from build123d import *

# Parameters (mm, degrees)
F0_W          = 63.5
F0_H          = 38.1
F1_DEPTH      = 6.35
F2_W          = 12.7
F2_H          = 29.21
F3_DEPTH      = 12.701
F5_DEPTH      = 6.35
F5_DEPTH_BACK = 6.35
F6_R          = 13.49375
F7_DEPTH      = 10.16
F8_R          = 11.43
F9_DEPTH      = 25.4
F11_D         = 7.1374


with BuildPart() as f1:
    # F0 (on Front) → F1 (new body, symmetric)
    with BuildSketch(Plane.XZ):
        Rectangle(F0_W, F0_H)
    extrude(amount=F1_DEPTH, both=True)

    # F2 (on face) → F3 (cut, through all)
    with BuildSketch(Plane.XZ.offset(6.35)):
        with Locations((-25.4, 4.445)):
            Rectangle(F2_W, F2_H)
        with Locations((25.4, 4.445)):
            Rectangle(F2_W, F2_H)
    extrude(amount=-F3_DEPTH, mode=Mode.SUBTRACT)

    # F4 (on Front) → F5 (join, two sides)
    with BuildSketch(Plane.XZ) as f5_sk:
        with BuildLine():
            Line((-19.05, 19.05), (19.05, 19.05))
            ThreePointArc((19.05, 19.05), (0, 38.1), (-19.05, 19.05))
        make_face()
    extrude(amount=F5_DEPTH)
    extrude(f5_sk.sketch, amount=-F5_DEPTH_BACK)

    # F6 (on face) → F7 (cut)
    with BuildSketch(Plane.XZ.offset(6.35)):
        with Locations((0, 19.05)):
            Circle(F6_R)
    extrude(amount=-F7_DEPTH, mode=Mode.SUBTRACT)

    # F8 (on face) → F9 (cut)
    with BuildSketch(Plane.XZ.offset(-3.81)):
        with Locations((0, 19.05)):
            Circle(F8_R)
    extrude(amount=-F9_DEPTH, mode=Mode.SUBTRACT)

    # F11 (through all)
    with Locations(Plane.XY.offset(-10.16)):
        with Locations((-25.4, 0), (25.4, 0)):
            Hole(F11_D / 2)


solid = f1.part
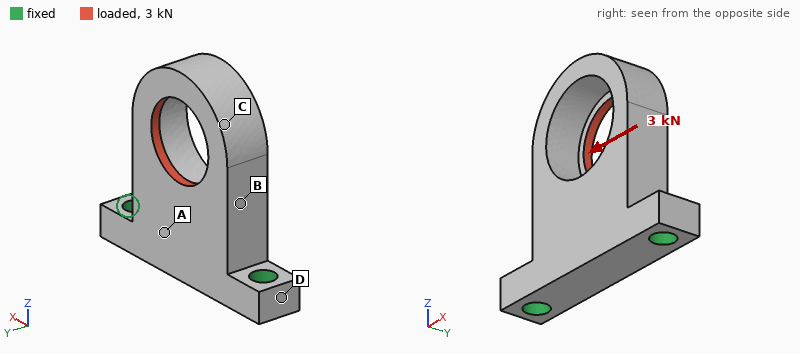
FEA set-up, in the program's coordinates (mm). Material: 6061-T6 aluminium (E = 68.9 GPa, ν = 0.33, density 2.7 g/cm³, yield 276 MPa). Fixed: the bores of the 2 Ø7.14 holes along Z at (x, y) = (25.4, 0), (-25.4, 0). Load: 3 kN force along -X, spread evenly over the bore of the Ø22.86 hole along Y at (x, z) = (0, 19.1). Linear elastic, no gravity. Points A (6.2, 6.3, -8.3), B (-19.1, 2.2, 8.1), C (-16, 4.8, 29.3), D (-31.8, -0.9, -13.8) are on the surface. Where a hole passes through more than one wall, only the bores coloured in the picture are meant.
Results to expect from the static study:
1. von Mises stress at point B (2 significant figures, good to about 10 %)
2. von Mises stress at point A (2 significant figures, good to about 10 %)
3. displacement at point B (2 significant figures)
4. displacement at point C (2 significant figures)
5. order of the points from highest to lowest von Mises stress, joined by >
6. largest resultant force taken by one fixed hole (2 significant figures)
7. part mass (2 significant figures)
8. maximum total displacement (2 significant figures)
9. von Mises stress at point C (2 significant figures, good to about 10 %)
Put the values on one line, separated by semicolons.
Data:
54 MPa; 21 MPa; 30 µm; 92 µm; B > C > A > D; 2.9 kN; 57 g; 98 µm; 41 MPa
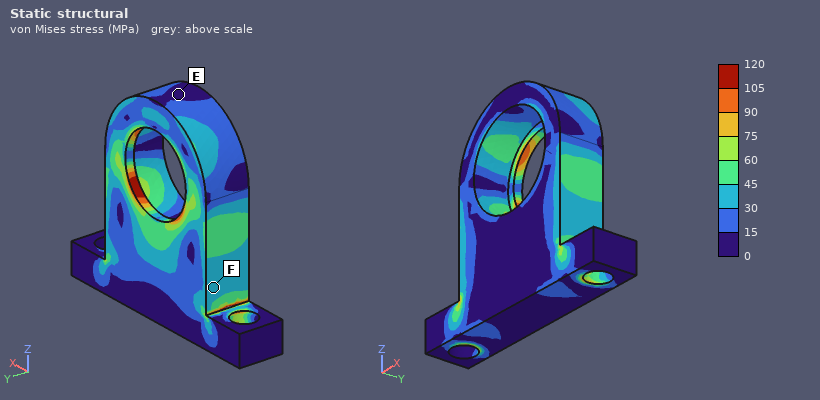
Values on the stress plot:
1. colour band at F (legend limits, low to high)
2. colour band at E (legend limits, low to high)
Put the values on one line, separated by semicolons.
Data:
30 to 45 MPa; 0 to 15 MPa
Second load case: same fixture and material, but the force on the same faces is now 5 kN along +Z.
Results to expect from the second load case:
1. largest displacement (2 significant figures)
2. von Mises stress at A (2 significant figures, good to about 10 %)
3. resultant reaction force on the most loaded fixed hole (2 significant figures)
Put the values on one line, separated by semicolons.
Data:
0.20 mm; 16 MPa; 2.7 kN
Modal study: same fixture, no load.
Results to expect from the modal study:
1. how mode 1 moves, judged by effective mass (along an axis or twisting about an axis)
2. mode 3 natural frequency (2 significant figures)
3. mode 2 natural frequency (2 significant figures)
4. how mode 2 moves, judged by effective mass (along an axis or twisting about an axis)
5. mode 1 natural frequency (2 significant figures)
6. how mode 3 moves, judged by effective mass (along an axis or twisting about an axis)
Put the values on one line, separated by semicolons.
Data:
along Y; 9000 Hz; 7000 Hz; along X; 2800 Hz; twisting about Z
